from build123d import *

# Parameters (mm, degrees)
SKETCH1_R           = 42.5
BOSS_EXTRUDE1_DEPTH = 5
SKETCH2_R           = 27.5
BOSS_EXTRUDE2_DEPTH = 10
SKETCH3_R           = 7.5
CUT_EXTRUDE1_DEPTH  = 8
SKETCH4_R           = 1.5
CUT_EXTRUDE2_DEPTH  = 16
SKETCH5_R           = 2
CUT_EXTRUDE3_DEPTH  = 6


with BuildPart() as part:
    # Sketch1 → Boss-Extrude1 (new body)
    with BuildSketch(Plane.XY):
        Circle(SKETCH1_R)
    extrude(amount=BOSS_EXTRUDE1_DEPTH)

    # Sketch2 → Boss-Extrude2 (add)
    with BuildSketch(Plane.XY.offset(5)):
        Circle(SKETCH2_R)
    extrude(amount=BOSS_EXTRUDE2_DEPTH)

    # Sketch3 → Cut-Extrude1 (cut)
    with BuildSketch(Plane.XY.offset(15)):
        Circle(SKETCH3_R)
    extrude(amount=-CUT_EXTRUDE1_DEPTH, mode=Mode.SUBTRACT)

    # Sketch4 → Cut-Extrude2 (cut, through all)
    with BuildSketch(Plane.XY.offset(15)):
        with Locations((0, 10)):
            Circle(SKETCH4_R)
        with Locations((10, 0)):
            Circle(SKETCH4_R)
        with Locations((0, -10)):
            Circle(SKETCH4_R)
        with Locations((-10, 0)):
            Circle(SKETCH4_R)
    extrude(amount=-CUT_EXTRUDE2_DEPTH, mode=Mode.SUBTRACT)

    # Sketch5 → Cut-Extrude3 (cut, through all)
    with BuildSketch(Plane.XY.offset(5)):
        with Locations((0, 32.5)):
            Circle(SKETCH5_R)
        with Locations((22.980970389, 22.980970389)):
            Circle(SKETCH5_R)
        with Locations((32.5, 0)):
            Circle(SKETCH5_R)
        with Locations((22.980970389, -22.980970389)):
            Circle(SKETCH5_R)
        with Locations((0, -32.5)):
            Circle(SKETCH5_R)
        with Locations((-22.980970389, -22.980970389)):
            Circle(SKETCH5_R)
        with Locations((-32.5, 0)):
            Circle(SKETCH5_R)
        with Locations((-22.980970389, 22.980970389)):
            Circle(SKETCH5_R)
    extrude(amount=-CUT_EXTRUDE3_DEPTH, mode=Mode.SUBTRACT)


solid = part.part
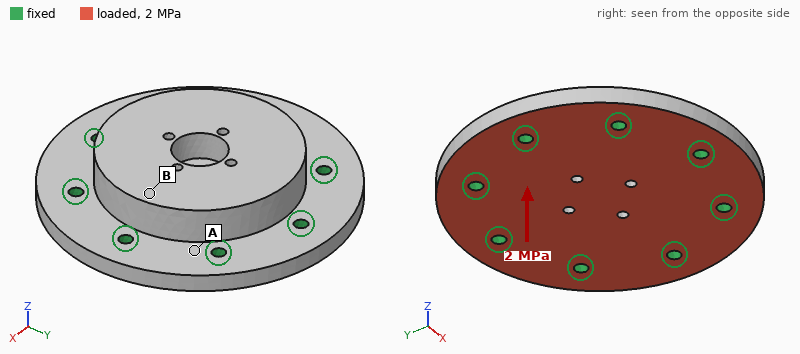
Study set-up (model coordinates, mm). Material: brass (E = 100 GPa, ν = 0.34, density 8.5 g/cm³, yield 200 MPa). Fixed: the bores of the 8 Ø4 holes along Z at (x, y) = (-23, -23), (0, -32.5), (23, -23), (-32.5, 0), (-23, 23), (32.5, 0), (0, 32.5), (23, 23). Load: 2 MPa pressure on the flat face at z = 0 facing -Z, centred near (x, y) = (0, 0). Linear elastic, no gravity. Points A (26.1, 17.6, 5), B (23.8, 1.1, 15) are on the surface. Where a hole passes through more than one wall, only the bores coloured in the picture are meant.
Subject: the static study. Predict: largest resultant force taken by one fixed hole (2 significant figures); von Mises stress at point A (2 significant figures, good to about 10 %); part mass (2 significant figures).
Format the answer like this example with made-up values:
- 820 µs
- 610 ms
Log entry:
- 1.4 kN
- 13 MPa
- 420 g
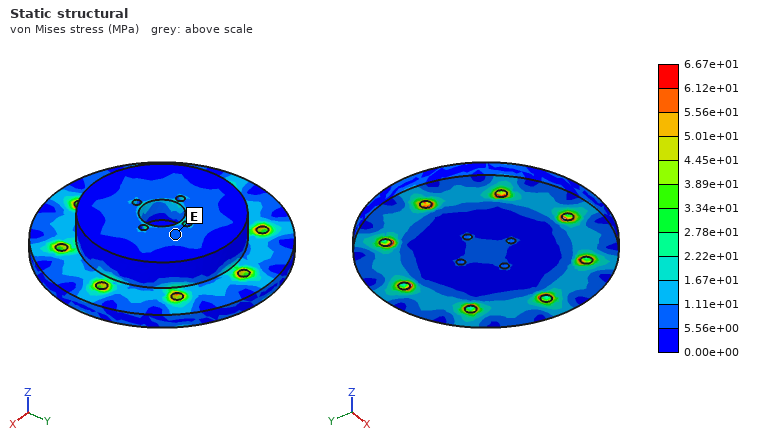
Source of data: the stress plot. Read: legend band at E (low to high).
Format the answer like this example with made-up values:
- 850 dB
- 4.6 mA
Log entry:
- 5.56e+00 to 1.11e+01 MPa
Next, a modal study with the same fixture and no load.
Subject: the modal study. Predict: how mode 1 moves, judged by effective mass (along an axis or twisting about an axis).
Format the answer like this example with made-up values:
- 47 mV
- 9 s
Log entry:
- along Z
